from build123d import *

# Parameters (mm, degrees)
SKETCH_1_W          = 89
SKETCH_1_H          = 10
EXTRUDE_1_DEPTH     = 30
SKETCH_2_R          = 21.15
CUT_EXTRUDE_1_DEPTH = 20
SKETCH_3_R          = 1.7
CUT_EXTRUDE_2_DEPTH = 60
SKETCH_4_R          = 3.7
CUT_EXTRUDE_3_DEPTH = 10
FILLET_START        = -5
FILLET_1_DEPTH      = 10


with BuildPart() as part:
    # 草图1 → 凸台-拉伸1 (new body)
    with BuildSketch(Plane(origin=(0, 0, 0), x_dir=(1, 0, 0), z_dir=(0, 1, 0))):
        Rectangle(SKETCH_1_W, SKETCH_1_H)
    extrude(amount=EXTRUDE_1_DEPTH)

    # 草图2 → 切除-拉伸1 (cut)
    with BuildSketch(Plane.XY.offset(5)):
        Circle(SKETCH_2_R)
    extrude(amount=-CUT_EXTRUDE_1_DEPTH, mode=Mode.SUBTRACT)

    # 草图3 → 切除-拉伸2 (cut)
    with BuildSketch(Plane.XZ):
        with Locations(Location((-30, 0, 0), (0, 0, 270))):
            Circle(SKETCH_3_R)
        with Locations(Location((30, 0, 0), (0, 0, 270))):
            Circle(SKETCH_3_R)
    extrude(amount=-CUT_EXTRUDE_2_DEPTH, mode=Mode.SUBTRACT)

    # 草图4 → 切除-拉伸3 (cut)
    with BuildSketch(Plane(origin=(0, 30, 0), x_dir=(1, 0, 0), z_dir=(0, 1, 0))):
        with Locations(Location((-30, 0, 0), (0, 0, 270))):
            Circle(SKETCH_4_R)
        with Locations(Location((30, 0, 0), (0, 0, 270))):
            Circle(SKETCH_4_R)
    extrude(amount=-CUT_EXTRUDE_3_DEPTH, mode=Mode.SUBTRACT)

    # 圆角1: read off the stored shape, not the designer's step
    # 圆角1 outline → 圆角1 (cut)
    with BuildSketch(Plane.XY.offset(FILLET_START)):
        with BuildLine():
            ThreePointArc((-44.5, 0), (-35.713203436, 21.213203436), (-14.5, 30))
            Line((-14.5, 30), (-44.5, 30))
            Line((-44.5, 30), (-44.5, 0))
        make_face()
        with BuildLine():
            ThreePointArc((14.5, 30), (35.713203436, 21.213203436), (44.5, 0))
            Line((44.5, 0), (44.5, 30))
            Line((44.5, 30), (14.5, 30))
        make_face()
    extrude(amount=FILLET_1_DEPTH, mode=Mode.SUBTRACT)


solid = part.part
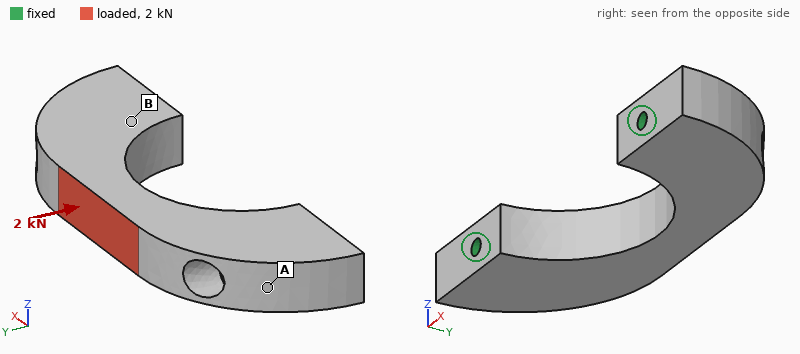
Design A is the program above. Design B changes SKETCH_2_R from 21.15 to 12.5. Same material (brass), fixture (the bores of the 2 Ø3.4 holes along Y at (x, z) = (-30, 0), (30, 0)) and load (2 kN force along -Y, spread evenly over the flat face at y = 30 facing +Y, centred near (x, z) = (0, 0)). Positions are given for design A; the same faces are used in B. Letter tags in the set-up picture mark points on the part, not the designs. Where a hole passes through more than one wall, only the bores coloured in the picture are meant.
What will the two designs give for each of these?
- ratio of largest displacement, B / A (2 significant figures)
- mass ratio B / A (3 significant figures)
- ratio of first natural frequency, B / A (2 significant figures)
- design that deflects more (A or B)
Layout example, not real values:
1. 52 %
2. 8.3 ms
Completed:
1. 0.56
2. 1.31
3. 0.94
4. A
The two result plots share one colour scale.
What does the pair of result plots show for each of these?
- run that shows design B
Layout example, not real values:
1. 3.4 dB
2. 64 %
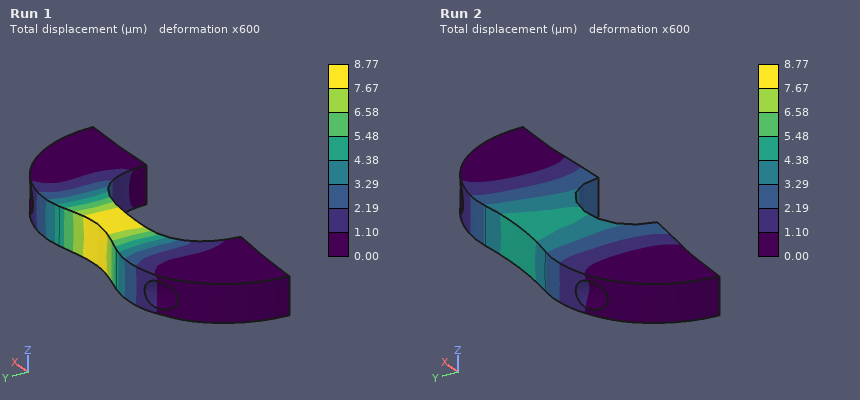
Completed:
1. Run 2
